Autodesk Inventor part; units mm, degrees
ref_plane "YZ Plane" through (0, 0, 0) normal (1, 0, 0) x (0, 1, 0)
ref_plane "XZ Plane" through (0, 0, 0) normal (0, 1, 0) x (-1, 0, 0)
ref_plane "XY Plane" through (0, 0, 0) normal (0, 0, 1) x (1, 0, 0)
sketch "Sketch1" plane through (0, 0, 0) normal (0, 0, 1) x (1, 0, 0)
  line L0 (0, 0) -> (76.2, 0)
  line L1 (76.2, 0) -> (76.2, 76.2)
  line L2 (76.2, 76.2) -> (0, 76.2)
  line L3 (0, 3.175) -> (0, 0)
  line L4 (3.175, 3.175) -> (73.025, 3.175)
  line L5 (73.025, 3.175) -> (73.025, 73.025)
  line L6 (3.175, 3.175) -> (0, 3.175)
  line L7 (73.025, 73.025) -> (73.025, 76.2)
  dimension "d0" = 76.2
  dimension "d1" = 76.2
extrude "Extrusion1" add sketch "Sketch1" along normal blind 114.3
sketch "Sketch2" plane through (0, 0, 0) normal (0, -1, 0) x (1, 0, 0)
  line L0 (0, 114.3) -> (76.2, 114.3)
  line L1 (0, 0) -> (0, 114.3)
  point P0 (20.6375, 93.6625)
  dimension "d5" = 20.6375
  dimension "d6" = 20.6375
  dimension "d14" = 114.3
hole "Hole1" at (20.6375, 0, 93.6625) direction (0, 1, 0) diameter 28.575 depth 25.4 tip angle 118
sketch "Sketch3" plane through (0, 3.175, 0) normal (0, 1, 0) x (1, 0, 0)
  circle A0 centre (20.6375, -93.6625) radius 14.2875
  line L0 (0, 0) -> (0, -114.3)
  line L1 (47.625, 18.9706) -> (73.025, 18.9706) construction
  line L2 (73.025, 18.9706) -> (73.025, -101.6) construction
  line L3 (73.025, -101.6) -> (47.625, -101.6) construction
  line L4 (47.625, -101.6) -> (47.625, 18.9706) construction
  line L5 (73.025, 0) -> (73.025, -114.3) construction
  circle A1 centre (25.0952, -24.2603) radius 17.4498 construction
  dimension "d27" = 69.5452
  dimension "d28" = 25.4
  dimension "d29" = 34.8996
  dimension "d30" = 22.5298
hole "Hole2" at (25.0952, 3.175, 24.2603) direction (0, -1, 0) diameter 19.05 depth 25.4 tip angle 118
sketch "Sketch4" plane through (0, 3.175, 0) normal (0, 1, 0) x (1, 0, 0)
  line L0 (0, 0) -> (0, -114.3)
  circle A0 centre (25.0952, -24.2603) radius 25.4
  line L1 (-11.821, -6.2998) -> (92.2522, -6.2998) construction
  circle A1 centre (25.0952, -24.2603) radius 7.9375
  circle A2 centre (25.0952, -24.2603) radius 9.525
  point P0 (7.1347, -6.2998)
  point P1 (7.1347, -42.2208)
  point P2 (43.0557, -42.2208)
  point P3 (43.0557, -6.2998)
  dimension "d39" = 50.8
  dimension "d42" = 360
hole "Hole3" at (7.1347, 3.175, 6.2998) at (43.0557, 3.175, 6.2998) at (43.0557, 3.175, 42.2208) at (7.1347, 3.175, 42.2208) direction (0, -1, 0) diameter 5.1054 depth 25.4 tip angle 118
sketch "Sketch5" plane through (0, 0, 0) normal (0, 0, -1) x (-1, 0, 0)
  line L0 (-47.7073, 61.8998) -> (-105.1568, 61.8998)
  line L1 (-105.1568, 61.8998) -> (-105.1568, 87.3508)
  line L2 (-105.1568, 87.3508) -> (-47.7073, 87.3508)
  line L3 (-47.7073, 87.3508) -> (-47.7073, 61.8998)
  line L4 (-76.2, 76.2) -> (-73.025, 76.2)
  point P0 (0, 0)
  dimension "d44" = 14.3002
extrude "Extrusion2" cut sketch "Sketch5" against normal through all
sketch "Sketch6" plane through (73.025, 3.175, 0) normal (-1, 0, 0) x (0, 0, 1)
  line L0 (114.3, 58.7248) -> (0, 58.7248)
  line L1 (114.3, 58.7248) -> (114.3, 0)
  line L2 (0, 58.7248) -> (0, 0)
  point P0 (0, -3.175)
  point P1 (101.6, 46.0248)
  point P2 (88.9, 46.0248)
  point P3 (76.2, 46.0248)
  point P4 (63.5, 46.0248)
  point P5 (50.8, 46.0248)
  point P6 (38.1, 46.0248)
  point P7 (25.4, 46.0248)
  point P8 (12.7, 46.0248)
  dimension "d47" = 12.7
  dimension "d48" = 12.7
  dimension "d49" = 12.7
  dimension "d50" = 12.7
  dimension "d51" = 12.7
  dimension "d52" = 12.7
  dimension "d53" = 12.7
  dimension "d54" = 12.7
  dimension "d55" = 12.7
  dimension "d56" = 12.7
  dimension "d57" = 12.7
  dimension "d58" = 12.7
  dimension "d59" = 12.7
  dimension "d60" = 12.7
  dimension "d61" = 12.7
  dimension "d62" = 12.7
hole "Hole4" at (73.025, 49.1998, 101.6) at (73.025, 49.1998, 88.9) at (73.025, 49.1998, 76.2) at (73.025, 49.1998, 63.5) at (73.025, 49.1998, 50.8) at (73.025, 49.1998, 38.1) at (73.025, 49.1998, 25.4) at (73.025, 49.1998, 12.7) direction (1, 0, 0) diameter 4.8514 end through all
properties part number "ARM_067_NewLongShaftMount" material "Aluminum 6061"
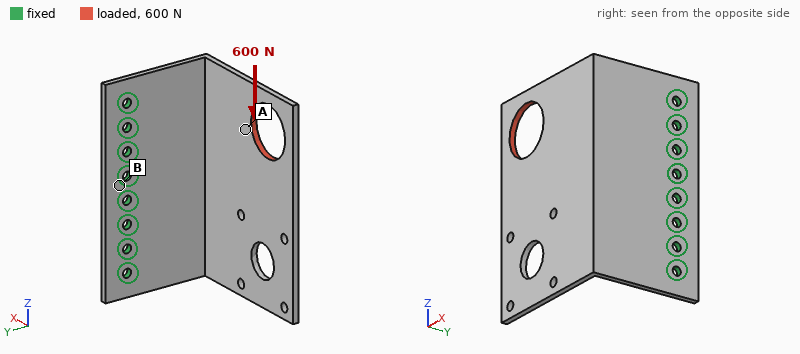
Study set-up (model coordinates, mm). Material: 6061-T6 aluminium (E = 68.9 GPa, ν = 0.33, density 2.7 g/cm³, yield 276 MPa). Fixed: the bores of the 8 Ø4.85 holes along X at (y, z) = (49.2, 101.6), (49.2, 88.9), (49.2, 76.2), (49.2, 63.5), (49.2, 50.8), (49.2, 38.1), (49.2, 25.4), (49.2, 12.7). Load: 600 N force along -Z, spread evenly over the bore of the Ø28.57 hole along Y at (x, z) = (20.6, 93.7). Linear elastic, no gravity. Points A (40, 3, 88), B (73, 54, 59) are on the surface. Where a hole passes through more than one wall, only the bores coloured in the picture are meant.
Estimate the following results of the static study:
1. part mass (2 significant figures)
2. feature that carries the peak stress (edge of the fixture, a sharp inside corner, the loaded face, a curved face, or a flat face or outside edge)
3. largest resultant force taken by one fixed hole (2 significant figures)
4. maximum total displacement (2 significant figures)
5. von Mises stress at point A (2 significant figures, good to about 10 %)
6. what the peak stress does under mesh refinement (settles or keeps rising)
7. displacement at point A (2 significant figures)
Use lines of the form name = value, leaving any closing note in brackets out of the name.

part mass = 120 g
feature that carries the peak stress = edge of the fixture
largest resultant force taken by one fixed hole = 380 N
maximum total displacement = 1.6 mm
von Mises stress at point A = 31 MPa
what the peak stress does under mesh refinement = keeps rising
displacement at point A = 0.77 mm
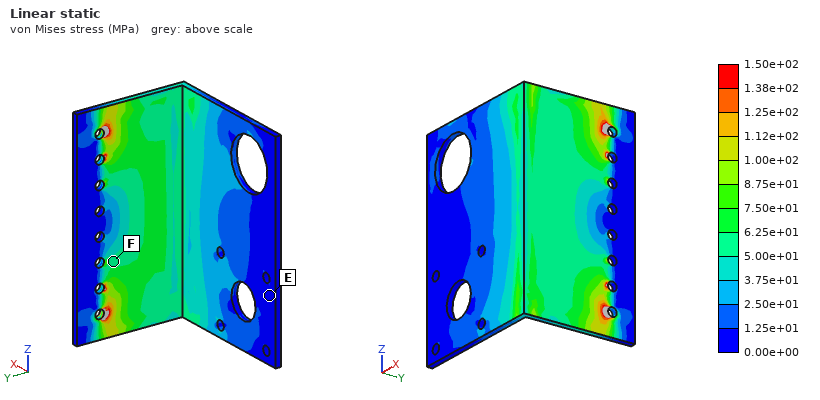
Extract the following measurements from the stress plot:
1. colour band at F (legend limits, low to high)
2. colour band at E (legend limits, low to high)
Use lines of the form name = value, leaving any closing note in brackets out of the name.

colour band at F = 5.00e+01 to 6.25e+01 MPa
colour band at E = 0.00e+00 to 1.25e+01 MPa
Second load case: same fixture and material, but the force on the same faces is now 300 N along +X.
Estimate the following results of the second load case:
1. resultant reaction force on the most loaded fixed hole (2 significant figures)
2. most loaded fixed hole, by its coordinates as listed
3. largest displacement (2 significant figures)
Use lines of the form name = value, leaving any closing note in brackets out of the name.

resultant reaction force on the most loaded fixed hole = 120 N
most loaded fixed hole, by its coordinates as listed = (49.2, 101.6)
largest displacement = 1.5 mm
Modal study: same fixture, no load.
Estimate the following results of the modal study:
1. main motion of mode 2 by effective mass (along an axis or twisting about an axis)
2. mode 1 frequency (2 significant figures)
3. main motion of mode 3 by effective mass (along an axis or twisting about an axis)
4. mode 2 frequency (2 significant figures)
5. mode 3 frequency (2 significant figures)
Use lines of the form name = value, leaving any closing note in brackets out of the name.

main motion of mode 2 by effective mass = along Z
mode 1 frequency = 260 Hz
main motion of mode 3 by effective mass = along X
mode 2 frequency = 490 Hz
mode 3 frequency = 760 Hz
